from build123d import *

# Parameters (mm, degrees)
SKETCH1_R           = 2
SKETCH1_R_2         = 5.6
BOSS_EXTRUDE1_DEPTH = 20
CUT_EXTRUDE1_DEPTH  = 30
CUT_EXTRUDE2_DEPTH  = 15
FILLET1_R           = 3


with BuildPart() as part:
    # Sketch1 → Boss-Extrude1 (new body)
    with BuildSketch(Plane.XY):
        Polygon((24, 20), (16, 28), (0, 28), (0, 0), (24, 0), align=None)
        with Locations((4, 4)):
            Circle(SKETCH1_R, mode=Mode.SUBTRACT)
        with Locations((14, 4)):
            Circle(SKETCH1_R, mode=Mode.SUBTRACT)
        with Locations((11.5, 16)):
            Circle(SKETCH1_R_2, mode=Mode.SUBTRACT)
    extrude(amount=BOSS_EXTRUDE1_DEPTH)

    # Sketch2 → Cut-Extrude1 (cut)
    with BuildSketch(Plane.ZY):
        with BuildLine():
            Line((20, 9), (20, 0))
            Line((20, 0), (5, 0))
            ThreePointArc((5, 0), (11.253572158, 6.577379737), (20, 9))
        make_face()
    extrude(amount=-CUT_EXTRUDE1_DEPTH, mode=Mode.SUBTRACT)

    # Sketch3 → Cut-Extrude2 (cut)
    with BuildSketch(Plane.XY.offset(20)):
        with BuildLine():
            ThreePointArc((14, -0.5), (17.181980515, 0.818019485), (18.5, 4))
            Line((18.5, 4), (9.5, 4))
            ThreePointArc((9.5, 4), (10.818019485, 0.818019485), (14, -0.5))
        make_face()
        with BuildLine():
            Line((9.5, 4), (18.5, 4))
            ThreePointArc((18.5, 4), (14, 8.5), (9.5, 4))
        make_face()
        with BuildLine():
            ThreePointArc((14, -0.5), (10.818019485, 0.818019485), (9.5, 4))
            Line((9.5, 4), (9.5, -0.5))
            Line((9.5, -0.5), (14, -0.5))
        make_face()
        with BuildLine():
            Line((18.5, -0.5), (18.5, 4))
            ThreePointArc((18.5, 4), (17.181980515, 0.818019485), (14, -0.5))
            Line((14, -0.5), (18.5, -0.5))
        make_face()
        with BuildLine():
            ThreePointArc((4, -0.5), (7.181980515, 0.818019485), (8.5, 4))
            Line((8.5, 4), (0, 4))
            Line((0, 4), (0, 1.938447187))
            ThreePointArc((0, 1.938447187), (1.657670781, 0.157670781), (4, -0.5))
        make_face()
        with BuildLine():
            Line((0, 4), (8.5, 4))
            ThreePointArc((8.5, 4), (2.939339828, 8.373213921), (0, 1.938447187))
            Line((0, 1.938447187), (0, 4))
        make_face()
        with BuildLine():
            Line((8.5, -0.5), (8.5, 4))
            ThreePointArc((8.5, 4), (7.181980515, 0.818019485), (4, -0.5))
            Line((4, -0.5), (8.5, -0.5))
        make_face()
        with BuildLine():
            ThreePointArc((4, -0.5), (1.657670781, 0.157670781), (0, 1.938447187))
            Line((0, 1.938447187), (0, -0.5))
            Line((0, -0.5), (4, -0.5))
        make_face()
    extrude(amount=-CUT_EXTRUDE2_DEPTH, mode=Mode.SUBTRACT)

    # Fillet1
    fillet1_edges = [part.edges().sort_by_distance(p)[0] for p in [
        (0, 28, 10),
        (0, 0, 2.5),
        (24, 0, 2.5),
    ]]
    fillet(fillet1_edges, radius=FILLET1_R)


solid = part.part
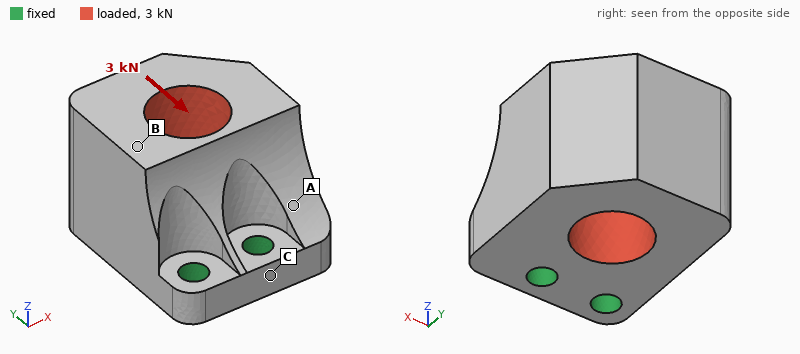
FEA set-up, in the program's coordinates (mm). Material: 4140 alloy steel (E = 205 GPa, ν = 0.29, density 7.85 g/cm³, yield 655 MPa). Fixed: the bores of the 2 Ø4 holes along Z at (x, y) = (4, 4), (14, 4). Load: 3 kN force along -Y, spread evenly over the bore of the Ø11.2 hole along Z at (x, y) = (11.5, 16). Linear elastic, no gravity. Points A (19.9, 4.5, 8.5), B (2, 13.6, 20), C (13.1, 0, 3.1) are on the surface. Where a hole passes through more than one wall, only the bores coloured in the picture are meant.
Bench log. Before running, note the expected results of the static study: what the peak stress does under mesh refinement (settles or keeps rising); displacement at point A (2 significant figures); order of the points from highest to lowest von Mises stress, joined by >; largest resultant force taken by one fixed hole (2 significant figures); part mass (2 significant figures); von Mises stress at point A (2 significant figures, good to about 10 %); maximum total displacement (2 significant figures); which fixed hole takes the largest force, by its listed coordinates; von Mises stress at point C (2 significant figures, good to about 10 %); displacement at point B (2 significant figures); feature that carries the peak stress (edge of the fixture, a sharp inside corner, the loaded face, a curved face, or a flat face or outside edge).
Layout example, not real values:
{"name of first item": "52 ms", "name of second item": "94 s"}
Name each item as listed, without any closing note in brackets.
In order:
{"what the peak stress does under mesh refinement": "keeps rising", "displacement at point A": "12 µm", "order of the points from highest to lowest von Mises stress, joined by >": "A > C > B", "largest resultant force taken by one fixed hole": "2.0 kN", "part mass": "62 g", "von Mises stress at point A": "95 MPa", "maximum total displacement": "55 µm", "which fixed hole takes the largest force, by its listed coordinates": "(14, 4)", "von Mises stress at point C": "46 MPa", "displacement at point B": "36 µm", "feature that carries the peak stress": "edge of the fixture"}
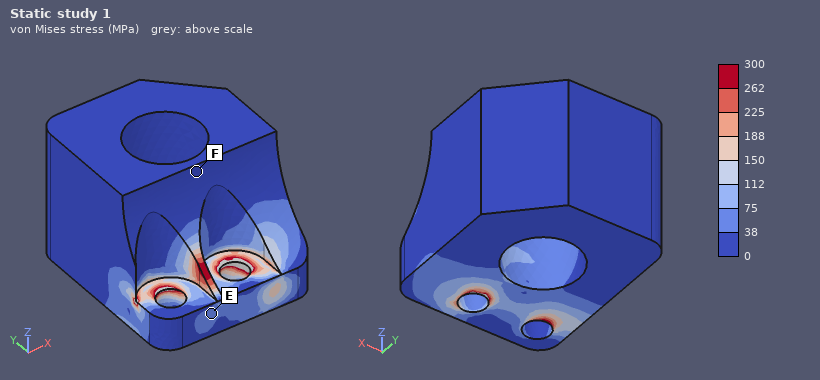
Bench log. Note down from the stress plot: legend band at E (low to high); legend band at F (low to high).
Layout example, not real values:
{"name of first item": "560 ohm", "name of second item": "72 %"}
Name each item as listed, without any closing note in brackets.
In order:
{"legend band at E": "38 to 75 MPa", "legend band at F": "0 to 38 MPa"}
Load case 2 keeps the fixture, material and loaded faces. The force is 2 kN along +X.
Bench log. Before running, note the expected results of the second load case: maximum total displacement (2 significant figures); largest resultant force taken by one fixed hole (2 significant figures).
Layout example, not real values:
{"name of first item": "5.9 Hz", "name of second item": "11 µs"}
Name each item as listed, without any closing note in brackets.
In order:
{"maximum total displacement": "16 µm", "largest resultant force taken by one fixed hole": "2.1 kN"}
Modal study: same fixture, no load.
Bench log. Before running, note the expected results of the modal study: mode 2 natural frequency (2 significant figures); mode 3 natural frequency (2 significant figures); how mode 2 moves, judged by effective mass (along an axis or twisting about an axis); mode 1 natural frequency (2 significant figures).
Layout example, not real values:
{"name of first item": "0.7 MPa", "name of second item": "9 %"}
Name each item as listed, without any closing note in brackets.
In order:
{"mode 2 natural frequency": "8900 Hz", "mode 3 natural frequency": "12 kHz", "how mode 2 moves, judged by effective mass": "along X", "mode 1 natural frequency": "4500 Hz"}
